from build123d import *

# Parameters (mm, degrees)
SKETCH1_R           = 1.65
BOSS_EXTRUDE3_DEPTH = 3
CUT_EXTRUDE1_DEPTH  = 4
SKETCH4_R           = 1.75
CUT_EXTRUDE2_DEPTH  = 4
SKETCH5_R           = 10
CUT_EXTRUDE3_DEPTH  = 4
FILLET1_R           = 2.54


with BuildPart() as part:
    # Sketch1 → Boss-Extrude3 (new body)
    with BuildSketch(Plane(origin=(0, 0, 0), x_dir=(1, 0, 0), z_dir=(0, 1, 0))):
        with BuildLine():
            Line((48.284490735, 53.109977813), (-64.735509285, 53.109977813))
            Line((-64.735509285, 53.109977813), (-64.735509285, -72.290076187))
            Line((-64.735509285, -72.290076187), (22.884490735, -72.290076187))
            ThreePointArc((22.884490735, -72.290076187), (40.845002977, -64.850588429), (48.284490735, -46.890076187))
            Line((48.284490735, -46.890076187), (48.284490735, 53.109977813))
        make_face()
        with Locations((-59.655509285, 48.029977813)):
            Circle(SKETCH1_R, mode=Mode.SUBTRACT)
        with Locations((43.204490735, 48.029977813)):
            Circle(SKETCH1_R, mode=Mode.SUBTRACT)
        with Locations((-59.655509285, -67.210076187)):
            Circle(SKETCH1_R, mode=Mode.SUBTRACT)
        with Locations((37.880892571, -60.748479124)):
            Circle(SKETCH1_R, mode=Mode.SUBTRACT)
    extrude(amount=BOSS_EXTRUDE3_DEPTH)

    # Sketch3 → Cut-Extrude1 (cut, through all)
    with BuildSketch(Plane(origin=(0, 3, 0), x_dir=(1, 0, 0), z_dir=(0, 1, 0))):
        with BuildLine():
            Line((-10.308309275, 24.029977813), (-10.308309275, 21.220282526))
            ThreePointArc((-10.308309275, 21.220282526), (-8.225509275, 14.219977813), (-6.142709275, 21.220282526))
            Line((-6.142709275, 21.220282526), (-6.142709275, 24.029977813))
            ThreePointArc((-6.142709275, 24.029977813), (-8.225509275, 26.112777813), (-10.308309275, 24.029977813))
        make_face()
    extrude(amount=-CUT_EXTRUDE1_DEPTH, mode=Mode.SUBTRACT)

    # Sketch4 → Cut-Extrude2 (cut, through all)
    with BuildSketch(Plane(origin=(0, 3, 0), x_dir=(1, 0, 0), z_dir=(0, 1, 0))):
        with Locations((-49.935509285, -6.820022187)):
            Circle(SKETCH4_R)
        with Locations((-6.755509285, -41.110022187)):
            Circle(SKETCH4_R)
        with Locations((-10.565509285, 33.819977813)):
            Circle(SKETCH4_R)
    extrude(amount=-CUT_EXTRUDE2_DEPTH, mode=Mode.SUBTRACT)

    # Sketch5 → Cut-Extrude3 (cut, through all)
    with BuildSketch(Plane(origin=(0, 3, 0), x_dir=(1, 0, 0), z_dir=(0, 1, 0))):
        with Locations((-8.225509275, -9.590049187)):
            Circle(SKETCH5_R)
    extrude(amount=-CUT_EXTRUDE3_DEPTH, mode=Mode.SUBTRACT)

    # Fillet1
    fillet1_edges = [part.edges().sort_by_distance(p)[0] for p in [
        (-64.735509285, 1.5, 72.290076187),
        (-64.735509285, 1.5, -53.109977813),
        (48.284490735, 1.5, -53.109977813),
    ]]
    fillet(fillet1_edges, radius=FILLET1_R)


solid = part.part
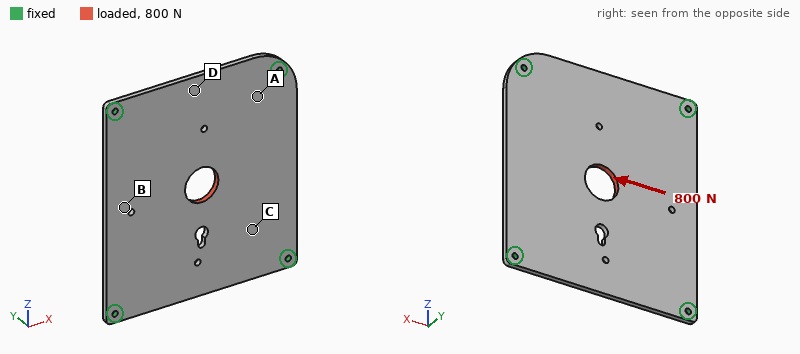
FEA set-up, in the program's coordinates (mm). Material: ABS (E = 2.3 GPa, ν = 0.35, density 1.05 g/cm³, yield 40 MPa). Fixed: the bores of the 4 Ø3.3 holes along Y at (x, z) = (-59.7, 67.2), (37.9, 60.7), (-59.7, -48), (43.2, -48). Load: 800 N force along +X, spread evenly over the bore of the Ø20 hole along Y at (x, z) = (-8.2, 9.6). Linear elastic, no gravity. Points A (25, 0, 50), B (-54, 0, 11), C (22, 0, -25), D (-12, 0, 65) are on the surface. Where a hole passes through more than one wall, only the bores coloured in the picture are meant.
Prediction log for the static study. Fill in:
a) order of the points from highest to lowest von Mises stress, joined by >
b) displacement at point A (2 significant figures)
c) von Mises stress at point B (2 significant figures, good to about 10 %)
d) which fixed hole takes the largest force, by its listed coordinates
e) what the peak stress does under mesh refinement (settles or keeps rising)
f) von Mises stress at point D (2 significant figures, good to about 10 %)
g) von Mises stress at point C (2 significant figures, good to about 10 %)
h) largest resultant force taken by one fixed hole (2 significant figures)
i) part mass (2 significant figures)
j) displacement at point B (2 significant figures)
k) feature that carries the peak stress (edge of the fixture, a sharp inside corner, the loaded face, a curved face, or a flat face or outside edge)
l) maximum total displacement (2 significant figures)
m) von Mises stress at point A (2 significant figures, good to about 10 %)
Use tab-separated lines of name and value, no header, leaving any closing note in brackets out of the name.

order of the points from highest to lowest von Mises stress, joined by >	A > C > B > D
displacement at point A	0.047 mm
von Mises stress at point B	1.4 MPa
which fixed hole takes the largest force, by its listed coordinates	(37.9, 60.7)
what the peak stress does under mesh refinement	keeps rising
von Mises stress at point D	0.71 MPa
von Mises stress at point C	2.7 MPa
largest resultant force taken by one fixed hole	260 N
part mass	43 g
displacement at point B	0.11 mm
feature that carries the peak stress	edge of the fixture
maximum total displacement	0.14 mm
von Mises stress at point A	3.6 MPa
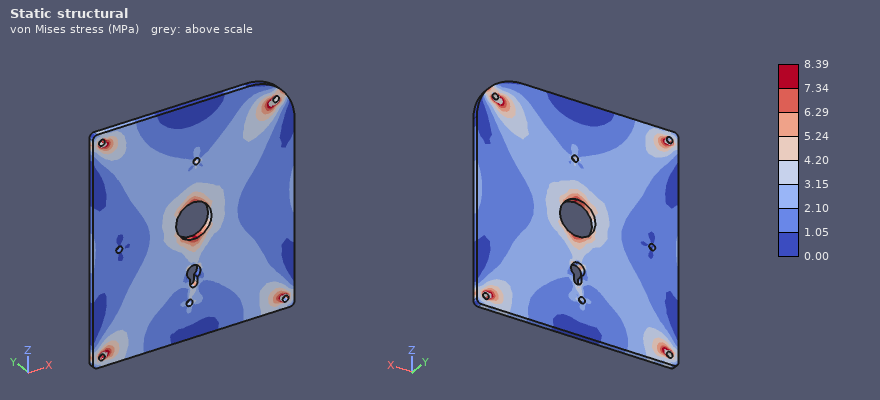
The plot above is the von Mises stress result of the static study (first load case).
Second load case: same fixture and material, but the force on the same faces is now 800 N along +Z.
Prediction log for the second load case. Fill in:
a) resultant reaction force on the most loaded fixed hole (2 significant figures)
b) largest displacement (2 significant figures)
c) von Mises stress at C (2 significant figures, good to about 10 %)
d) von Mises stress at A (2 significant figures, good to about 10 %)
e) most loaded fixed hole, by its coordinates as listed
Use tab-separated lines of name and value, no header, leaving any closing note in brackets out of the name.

resultant reaction force on the most loaded fixed hole	250 N
largest displacement	0.12 mm
von Mises stress at C	2.4 MPa
von Mises stress at A	3.2 MPa
most loaded fixed hole, by its coordinates as listed	(37.9, 60.7)
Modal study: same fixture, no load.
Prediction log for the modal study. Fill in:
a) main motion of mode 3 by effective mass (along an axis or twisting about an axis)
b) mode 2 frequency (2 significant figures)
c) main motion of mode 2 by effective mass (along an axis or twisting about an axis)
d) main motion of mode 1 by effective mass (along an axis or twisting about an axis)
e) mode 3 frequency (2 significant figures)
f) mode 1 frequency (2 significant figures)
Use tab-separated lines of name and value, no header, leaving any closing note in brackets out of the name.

main motion of mode 3 by effective mass	twisting about X
mode 2 frequency	400 Hz
main motion of mode 2 by effective mass	twisting about Z
main motion of mode 1 by effective mass	along Y
mode 3 frequency	450 Hz
mode 1 frequency	240 Hz
